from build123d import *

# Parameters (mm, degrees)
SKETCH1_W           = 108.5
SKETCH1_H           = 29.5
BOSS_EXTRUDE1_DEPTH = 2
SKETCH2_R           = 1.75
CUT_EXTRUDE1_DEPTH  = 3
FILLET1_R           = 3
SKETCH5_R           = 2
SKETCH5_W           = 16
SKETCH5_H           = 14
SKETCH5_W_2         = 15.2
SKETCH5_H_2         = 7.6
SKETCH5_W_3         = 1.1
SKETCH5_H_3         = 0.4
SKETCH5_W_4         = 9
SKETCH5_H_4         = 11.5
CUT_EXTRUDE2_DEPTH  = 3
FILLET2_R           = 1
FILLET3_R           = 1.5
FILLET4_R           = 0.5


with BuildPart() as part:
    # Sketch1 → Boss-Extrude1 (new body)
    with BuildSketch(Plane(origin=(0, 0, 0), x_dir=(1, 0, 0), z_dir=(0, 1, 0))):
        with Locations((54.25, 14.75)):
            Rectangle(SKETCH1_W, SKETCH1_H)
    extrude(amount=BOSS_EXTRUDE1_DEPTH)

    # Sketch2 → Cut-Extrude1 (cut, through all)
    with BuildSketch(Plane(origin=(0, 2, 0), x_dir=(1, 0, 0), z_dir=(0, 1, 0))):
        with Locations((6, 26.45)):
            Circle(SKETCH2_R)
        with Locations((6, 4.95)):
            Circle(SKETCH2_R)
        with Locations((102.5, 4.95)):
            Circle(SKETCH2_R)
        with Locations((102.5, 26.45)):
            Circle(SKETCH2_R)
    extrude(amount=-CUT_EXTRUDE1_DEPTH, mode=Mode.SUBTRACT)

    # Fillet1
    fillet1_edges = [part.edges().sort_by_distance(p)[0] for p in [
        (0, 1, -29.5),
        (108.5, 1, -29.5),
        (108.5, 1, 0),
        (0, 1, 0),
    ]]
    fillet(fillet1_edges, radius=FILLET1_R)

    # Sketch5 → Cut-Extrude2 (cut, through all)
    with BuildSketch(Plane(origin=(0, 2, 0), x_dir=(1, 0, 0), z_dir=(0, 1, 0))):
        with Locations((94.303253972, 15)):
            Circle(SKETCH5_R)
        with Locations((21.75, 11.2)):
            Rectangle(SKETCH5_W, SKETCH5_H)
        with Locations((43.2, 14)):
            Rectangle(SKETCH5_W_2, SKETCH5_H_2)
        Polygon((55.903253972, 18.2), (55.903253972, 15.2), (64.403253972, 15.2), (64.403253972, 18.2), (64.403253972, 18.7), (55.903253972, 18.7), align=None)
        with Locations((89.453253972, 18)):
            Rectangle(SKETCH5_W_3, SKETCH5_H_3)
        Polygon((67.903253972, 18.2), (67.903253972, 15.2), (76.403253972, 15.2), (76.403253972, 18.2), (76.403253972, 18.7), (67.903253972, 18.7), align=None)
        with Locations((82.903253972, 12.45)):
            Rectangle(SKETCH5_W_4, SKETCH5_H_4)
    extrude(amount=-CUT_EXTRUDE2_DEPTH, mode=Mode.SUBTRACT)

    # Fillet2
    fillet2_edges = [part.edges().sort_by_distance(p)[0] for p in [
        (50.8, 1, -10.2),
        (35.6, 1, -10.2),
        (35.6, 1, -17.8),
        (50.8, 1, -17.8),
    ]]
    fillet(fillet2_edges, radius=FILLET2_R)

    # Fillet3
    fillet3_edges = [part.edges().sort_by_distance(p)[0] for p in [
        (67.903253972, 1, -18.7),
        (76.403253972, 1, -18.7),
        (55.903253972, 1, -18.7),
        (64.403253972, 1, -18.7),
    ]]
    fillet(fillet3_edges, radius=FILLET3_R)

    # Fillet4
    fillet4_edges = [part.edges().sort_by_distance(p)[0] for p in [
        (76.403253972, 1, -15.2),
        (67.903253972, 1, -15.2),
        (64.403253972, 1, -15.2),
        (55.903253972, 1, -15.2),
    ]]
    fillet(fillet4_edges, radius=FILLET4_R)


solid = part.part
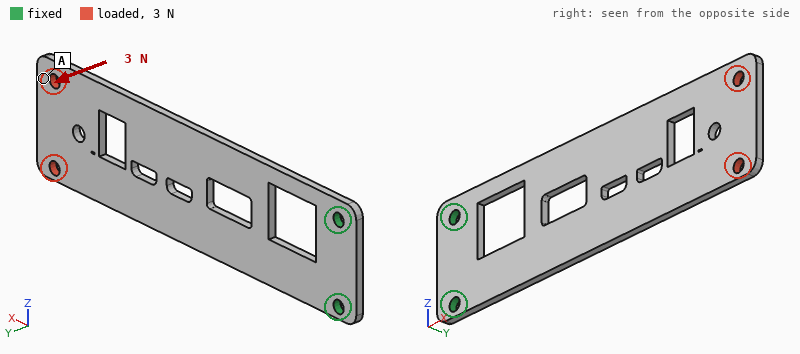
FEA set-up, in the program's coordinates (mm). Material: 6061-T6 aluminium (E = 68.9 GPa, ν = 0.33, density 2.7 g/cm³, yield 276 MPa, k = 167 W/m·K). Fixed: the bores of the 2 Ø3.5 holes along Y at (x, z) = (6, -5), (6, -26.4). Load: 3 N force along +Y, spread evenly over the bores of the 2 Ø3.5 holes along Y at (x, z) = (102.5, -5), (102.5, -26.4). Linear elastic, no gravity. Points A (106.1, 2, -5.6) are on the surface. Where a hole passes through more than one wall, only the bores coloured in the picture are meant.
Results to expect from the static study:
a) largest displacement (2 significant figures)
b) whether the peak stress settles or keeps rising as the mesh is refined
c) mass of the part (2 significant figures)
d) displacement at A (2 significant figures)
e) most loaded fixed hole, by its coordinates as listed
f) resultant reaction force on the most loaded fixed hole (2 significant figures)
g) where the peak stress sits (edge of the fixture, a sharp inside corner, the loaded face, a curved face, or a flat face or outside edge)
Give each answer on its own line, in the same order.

1.1 mm
keeps rising
14 g
1.1 mm
(6, -26.4)
2.1 N
edge of the fixture
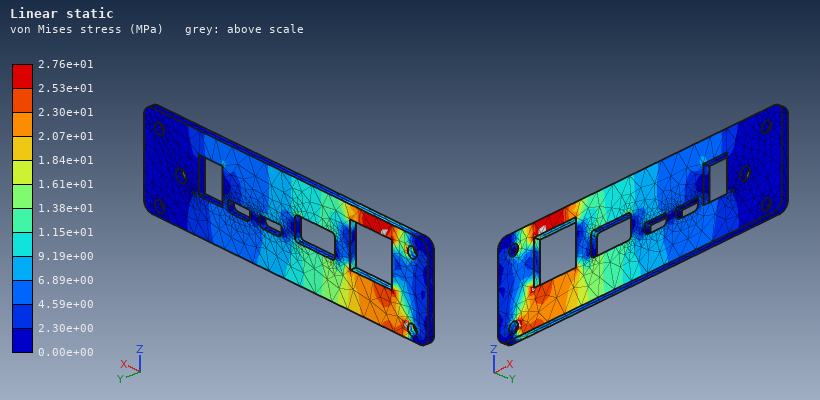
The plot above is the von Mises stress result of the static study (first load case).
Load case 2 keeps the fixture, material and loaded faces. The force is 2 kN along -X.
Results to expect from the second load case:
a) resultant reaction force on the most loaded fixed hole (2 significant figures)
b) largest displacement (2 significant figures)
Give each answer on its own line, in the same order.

1.0 kN
93 µm
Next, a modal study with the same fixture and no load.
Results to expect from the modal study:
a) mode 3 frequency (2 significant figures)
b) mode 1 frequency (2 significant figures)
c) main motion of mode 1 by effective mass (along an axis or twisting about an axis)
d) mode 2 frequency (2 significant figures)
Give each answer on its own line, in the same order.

950 Hz
130 Hz
along Y
910 Hz
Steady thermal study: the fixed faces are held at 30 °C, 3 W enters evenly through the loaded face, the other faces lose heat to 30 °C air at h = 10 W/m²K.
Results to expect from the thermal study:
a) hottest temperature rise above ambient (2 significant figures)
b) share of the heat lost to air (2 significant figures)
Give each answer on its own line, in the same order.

33 K
34 %
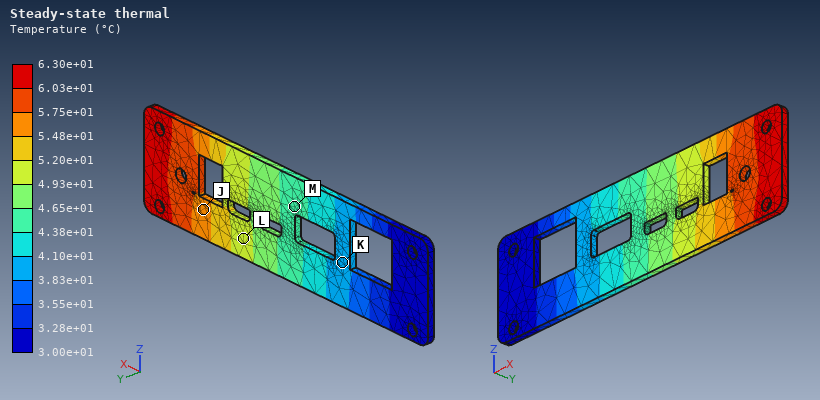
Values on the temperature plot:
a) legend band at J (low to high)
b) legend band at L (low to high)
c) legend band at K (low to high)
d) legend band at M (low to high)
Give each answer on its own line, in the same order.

5.48e+01 to 5.75e+01 °C
4.93e+01 to 5.20e+01 °C
3.83e+01 to 4.10e+01 °C
4.38e+01 to 4.65e+01 °C
